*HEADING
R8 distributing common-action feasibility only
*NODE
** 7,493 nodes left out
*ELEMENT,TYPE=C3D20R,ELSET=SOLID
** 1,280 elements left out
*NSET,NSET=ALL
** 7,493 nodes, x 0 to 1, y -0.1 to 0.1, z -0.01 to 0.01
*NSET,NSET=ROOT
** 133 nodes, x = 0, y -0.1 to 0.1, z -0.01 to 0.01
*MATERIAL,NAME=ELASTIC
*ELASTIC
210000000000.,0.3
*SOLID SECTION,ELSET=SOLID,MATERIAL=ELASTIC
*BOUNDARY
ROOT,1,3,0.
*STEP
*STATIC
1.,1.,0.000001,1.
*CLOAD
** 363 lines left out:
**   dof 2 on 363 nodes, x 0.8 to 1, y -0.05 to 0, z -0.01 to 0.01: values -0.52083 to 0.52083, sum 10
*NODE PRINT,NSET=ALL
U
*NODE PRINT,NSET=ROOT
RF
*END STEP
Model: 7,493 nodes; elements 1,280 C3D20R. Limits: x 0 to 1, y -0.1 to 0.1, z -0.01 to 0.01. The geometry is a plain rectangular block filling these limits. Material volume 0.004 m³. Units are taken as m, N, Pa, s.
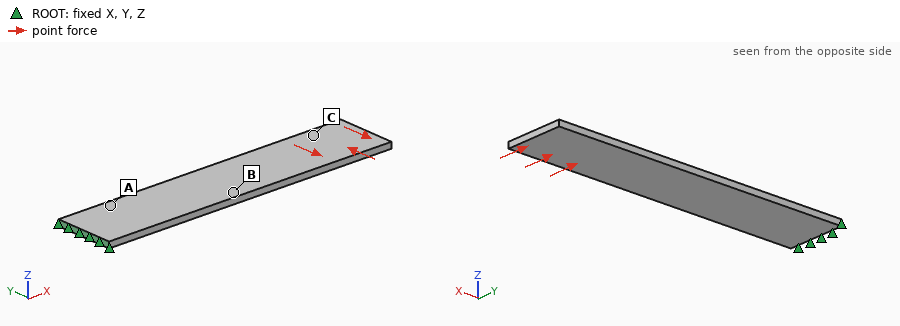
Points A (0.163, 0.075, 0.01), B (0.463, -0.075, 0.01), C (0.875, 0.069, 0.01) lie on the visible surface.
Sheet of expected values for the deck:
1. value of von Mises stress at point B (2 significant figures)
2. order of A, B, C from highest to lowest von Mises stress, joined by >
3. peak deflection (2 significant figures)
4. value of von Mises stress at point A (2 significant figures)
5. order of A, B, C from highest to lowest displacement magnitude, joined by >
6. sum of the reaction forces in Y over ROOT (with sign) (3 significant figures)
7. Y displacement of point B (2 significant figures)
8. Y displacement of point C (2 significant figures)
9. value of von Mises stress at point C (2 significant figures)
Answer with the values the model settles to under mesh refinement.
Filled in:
44000 Pa
A > B > C
1.6e-06 m
54000 Pa
C > B > A
-10.0 N
3.5e-07 m
9.6e-07 m
23000 Pa
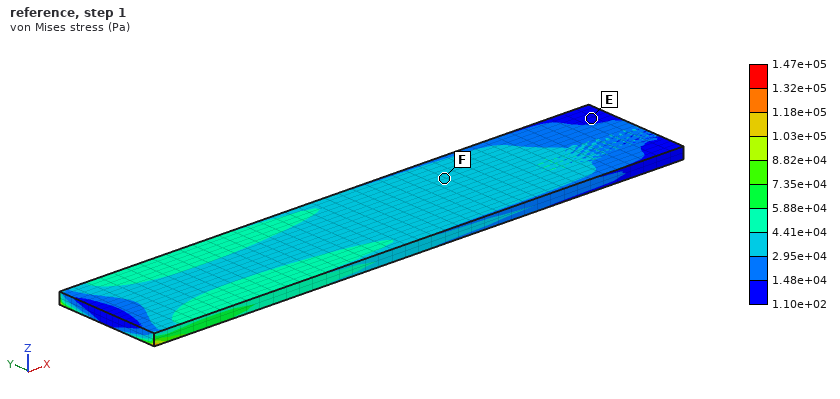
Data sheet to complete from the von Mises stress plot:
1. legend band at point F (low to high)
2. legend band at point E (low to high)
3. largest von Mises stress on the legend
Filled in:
2.95e+04 to 4.41e+04 Pa
1.10e+02 to 1.48e+04 Pa
1.47e+05 Pa
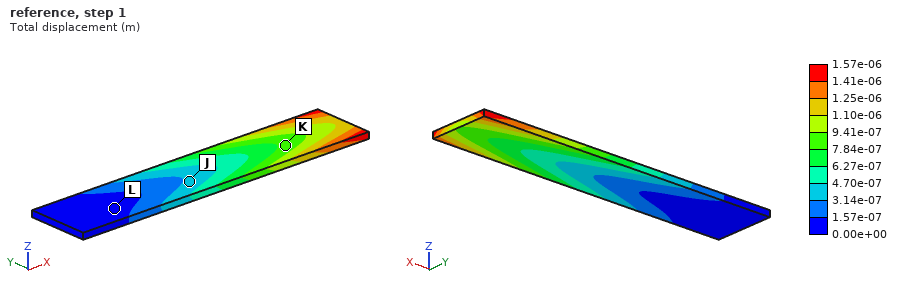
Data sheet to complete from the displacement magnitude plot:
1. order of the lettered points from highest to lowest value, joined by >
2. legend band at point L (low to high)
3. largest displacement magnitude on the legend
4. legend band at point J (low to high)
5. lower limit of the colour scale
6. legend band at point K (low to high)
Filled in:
K > J > L
0.00e+00 to 1.57e-07 m
1.57e-06 m
3.14e-07 to 4.70e-07 m
0.00e+00 m
7.84e-07 to 9.41e-07 m
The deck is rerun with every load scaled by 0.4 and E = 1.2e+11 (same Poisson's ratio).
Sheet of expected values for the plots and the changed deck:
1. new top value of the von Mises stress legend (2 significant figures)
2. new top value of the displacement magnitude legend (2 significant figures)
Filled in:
59000 Pa
1.1e-06 m
